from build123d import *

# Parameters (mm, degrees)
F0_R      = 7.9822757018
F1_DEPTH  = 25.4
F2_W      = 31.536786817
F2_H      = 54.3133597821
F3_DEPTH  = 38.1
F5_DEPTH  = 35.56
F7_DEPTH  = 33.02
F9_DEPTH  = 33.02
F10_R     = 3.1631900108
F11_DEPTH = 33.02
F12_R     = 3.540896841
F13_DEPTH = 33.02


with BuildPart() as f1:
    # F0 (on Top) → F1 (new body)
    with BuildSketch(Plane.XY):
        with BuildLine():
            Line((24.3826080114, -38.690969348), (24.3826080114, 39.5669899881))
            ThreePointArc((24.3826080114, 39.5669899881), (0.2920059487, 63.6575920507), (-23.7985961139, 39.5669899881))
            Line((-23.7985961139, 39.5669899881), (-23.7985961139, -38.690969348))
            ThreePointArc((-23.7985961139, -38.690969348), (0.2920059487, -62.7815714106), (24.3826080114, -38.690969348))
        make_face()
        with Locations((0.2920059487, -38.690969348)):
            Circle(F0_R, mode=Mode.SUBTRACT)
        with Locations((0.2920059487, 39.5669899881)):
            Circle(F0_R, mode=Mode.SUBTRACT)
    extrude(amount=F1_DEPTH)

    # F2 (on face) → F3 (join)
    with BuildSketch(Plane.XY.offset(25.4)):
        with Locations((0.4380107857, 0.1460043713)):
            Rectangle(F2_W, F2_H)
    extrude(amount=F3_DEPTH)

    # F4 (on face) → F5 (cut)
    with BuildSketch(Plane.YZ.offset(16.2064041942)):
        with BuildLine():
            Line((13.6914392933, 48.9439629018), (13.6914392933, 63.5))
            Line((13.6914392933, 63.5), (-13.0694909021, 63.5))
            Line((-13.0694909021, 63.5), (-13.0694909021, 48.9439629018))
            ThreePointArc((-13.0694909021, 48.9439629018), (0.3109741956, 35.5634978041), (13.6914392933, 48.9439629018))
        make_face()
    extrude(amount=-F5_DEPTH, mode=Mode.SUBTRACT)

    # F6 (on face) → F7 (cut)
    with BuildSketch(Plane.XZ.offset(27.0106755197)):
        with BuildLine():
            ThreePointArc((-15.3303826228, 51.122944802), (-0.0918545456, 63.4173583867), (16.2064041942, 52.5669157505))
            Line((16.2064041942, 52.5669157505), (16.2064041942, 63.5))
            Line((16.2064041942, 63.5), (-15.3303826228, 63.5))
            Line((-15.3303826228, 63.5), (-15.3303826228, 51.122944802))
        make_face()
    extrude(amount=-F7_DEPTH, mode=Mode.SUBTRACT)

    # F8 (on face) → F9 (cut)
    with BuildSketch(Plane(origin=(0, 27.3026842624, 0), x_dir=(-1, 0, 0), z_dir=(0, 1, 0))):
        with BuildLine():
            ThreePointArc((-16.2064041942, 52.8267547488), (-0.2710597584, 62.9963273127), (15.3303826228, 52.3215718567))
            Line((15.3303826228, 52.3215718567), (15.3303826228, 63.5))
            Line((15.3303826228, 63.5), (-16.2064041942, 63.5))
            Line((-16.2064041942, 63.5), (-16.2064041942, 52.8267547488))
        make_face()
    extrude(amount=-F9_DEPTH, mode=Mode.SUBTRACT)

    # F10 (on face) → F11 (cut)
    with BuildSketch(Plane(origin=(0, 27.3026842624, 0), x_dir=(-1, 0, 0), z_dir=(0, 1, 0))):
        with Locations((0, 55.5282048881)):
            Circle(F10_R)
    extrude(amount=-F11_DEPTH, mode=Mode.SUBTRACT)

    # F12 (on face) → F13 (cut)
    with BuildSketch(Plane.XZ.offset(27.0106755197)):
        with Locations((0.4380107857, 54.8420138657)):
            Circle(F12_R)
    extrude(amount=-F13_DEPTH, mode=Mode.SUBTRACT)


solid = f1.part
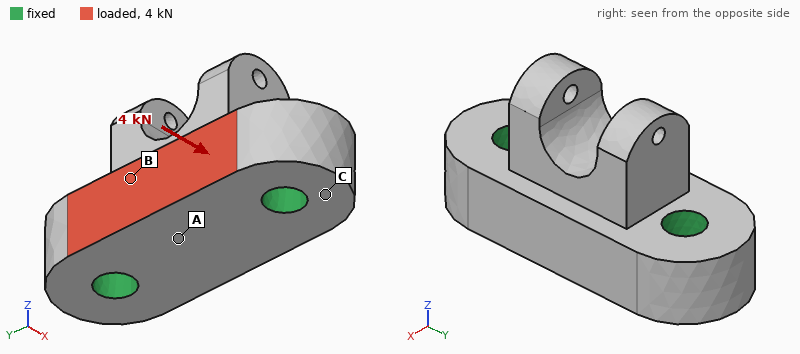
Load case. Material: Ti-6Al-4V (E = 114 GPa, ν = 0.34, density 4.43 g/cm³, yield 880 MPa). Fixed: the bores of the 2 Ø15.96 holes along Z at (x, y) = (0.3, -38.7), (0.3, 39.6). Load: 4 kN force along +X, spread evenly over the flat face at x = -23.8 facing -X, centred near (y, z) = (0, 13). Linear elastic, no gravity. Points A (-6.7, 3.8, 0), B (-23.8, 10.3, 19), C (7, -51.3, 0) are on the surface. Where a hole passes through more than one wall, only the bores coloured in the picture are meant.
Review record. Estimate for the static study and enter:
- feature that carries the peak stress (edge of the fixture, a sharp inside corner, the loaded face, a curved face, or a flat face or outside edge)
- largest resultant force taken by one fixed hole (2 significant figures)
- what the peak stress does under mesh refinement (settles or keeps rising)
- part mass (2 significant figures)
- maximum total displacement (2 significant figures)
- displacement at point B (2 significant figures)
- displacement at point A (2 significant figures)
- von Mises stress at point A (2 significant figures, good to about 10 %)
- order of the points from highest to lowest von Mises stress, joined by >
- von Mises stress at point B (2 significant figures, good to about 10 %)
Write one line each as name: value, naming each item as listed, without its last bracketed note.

feature that carries the peak stress: edge of the fixture
largest resultant force taken by one fixed hole: 2.0 kN
what the peak stress does under mesh refinement: keeps rising
part mass: 760 g
maximum total displacement: 1.3 µm
displacement at point B: 1.0 µm
displacement at point A: 1.1 µm
von Mises stress at point A: 1.4 MPa
order of the points from highest to lowest von Mises stress, joined by >: B > A > C
von Mises stress at point B: 2.3 MPa
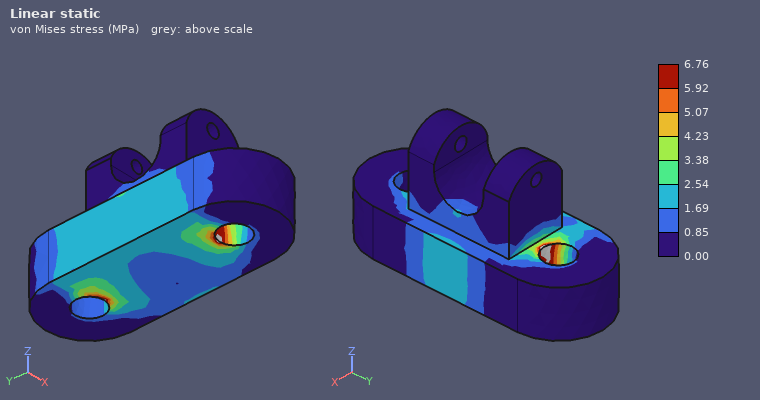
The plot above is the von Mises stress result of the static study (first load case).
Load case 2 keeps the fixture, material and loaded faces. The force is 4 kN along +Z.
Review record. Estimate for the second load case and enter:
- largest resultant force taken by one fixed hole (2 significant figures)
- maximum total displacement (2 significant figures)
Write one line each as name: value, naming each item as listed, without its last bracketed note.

largest resultant force taken by one fixed hole: 2.0 kN
maximum total displacement: 4.7 µm
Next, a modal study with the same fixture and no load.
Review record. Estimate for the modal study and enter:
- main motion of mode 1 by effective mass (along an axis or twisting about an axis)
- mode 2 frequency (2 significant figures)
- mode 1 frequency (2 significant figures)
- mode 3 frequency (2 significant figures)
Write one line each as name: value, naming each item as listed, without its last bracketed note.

main motion of mode 1 by effective mass: along X
mode 2 frequency: 12 kHz
mode 1 frequency: 8500 Hz
mode 3 frequency: 12 kHz
